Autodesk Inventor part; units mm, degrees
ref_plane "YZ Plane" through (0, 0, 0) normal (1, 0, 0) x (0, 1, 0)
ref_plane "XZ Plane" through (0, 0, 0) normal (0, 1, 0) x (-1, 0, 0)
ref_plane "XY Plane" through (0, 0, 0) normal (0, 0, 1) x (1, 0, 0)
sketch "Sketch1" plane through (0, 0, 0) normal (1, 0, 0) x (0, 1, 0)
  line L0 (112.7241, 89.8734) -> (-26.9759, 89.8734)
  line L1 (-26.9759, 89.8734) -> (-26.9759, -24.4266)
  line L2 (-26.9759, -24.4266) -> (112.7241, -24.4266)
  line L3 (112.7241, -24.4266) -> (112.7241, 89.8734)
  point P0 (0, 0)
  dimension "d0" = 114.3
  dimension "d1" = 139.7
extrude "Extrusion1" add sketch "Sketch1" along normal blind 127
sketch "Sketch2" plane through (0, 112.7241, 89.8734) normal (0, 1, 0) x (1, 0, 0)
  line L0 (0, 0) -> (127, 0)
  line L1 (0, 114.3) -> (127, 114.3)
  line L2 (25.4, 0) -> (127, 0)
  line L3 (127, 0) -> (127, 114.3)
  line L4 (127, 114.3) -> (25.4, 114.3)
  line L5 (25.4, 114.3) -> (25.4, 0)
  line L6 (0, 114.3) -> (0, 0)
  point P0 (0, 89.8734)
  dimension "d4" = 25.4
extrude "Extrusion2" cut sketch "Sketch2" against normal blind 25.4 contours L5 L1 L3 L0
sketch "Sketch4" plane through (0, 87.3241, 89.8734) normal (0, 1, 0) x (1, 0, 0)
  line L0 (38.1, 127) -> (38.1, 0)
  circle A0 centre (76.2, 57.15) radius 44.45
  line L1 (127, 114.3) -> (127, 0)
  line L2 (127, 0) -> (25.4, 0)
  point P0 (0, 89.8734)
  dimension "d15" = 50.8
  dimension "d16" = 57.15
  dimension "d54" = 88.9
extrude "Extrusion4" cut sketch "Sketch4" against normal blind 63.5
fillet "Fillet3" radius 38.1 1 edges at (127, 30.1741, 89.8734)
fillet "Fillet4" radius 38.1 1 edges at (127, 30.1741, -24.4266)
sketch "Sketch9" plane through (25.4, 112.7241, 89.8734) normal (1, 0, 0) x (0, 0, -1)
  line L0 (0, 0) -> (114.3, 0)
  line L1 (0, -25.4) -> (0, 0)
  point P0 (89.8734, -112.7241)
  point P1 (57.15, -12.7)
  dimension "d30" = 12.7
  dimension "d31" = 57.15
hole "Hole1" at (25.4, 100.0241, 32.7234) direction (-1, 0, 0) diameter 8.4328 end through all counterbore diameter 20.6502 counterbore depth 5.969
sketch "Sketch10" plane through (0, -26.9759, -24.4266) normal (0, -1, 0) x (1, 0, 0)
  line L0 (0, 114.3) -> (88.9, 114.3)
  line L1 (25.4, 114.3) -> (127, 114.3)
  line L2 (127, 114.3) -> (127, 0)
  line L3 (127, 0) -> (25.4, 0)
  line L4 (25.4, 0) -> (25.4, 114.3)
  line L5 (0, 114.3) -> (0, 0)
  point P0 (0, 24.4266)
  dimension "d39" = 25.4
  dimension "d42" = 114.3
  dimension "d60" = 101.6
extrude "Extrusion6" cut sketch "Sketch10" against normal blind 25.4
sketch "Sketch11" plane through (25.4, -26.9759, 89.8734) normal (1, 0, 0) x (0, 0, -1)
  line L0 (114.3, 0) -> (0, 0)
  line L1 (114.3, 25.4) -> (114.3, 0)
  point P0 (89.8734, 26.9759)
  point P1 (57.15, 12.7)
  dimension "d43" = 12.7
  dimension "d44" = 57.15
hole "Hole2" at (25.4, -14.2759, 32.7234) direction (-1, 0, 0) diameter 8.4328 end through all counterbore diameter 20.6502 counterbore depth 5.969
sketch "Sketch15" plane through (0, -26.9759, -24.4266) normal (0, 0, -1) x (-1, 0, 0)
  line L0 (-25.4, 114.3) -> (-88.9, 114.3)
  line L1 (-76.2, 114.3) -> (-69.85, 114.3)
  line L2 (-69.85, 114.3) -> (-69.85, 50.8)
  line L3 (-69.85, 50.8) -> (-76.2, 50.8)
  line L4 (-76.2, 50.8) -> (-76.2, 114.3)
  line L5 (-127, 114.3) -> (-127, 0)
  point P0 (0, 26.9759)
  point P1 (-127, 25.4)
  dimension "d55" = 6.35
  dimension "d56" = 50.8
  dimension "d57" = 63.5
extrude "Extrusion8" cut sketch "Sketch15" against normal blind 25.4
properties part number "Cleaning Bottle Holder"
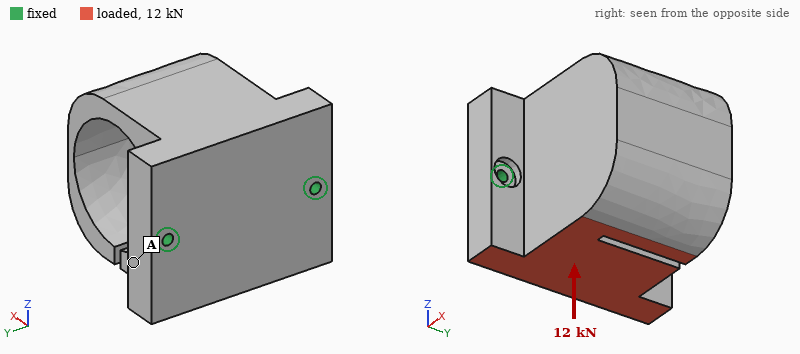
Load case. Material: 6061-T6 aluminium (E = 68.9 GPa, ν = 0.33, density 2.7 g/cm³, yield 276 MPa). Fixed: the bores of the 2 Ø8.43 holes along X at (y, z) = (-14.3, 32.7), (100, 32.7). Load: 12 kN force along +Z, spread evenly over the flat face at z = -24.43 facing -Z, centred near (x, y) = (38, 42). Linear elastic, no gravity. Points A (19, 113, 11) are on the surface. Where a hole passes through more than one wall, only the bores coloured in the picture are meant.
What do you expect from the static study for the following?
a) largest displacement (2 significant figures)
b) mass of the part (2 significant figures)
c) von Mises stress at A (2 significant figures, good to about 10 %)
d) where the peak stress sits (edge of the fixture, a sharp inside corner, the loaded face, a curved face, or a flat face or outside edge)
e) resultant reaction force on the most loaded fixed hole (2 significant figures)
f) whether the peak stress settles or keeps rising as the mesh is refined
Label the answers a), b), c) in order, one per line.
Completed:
a) 0.15 mm
b) 2.6 kg
c) 11 MPa
d) edge of the fixture
e) 6.1 kN
f) keeps rising
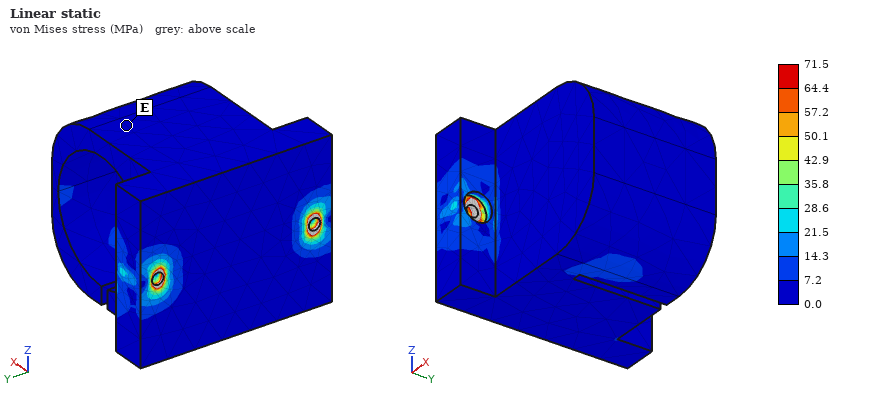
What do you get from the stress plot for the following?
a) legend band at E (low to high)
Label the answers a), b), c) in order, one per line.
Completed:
a) 0.0 to 7.2 MPa
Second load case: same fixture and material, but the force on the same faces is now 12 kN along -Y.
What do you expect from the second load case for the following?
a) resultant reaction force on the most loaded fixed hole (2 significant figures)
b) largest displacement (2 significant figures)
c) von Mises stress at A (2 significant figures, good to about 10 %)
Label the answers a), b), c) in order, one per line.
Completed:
a) 9.0 kN
b) 40 µm
c) 3.4 MPa
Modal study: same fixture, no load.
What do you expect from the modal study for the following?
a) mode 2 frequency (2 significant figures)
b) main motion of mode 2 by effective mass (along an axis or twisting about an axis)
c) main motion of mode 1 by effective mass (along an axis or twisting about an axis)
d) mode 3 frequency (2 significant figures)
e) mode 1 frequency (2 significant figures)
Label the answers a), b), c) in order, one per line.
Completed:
a) 1900 Hz
b) along Y
c) along Z
d) 2900 Hz
e) 830 Hz
